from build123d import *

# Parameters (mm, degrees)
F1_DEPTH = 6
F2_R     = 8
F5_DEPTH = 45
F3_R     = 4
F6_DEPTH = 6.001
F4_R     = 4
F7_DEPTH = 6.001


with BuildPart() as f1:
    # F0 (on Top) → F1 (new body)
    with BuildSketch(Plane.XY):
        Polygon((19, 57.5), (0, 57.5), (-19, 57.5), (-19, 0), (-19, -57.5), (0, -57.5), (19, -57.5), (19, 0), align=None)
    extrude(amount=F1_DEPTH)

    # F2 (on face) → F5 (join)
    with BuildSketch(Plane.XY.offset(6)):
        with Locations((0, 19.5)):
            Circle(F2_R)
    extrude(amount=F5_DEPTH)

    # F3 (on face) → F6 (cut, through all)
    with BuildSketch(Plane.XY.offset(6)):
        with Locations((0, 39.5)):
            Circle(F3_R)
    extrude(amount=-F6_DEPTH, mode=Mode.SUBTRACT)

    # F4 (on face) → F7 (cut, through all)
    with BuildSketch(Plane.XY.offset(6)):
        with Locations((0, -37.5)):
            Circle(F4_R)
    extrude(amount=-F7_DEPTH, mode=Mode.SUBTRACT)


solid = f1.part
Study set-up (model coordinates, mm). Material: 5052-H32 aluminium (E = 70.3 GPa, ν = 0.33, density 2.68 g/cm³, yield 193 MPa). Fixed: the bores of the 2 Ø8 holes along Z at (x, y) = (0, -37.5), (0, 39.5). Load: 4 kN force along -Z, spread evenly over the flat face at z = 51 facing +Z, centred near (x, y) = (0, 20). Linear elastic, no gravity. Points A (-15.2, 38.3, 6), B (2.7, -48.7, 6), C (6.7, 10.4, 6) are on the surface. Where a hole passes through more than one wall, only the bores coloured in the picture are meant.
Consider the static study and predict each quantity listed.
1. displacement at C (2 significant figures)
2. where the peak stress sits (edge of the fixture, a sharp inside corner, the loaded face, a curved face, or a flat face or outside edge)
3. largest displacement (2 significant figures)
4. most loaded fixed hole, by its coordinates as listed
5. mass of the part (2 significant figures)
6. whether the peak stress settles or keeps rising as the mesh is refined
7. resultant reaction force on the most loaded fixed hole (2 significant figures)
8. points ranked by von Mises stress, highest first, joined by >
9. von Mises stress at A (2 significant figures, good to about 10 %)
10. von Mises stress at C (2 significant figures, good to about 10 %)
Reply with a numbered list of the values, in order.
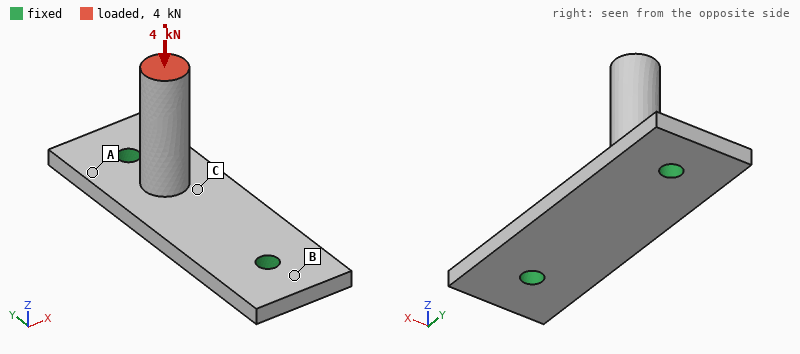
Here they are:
1. 0.11 mm
2. edge of the fixture
3. 0.23 mm
4. (0, 39.5)
5. 93 g
6. keeps rising
7. 3.3 kN
8. C > A > B
9. 43 MPa
10. 76 MPa
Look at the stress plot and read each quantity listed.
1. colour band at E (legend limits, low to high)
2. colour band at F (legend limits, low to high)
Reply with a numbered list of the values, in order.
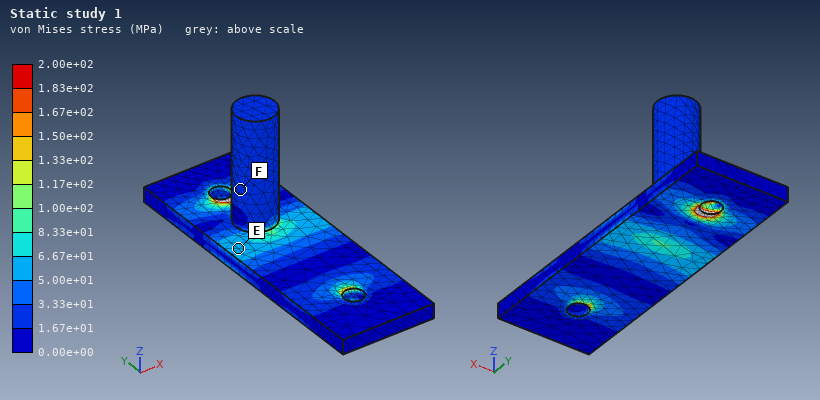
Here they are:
1. 5.00e+01 to 6.67e+01 MPa
2. 1.67e+01 to 3.33e+01 MPa
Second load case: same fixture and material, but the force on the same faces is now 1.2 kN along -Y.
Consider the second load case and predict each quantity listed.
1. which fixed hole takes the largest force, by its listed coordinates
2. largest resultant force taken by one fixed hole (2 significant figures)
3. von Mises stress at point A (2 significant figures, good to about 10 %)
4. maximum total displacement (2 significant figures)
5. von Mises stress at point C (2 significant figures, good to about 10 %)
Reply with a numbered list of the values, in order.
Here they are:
1. (0, 39.5)
2. 1.2 kN
3. 33 MPa
4. 0.48 mm
5. 96 MPa
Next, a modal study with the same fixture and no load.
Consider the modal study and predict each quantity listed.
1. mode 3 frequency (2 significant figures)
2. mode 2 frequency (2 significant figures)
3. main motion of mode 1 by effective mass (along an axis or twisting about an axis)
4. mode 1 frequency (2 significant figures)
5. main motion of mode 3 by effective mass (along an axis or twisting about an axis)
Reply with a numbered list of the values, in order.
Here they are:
1. 6200 Hz
2. 2600 Hz
3. along X
4. 2400 Hz
5. along Z
